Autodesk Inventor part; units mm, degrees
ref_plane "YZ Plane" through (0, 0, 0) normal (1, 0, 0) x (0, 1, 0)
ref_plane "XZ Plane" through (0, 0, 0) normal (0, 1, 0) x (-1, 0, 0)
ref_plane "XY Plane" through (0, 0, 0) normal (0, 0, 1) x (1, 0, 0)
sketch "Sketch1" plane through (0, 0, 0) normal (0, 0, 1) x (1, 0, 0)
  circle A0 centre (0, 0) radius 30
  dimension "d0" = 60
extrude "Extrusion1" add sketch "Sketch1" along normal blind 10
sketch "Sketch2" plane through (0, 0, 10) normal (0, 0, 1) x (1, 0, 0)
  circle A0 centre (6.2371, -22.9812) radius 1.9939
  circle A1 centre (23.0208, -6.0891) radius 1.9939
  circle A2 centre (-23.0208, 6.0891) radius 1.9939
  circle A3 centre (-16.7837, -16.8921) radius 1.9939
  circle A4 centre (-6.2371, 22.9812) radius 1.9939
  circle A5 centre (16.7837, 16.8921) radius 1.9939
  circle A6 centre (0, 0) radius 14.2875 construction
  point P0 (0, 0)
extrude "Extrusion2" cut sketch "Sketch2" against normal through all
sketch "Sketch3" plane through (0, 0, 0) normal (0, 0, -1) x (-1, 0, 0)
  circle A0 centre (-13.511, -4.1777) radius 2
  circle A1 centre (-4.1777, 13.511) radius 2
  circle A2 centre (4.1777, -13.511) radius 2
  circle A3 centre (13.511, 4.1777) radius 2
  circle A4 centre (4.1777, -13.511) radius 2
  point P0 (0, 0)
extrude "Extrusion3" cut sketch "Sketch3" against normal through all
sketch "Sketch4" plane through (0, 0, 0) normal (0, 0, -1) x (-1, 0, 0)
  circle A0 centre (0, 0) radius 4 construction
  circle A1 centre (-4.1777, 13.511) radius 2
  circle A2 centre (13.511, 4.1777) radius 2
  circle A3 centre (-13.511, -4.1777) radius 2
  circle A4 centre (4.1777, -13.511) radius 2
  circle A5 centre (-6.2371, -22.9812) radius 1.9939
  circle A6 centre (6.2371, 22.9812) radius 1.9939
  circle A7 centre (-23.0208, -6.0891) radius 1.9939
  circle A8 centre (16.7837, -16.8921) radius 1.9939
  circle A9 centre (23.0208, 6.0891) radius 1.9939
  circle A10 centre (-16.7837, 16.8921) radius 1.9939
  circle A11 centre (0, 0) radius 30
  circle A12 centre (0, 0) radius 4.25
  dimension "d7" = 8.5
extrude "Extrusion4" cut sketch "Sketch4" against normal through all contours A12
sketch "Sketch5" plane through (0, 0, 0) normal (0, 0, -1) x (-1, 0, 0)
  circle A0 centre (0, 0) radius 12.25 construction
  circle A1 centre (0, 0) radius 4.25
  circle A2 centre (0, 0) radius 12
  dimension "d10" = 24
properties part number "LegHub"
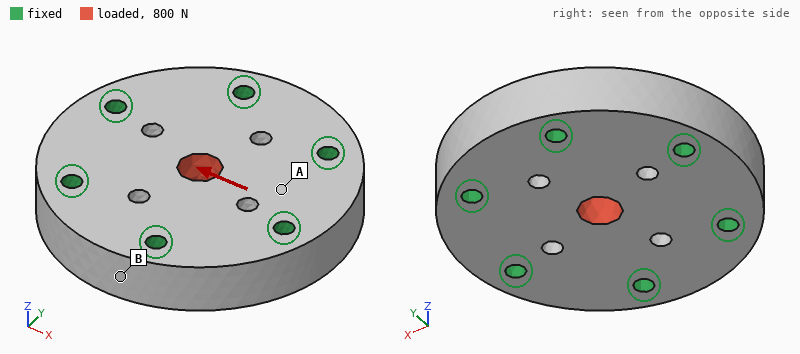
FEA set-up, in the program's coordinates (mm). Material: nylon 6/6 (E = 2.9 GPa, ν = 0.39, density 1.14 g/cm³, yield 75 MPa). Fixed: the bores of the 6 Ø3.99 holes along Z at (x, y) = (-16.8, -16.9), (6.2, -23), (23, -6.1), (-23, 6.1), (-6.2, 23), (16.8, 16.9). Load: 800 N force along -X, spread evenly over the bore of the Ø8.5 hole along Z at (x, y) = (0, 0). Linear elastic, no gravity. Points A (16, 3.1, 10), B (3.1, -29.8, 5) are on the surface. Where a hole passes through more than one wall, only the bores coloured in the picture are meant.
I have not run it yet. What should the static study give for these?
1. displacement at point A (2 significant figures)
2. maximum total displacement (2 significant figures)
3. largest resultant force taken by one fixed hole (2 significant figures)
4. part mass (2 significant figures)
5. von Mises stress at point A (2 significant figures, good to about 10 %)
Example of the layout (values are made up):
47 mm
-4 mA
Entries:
7.0 µm
16 µm
200 N
30 g
0.94 MPa
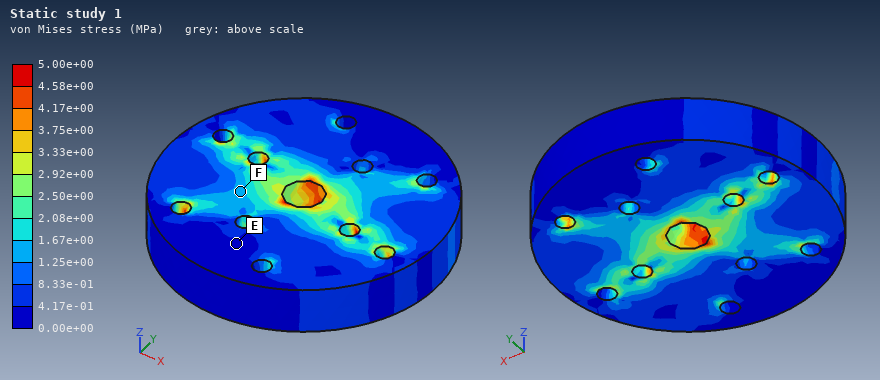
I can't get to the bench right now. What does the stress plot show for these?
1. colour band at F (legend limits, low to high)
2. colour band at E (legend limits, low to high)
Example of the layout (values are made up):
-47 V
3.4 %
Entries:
1.25e+00 to 1.67e+00 MPa
0.00e+00 to 4.17e-01 MPa
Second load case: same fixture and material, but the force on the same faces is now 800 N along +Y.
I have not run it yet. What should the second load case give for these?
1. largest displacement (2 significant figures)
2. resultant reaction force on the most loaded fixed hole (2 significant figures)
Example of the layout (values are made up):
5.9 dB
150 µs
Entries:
15 µm
210 N
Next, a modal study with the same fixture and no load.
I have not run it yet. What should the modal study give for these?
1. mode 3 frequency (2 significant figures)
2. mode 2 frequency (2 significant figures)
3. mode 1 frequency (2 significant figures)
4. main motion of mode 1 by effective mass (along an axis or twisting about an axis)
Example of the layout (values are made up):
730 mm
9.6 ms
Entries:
14 kHz
14 kHz
8600 Hz
along Z
